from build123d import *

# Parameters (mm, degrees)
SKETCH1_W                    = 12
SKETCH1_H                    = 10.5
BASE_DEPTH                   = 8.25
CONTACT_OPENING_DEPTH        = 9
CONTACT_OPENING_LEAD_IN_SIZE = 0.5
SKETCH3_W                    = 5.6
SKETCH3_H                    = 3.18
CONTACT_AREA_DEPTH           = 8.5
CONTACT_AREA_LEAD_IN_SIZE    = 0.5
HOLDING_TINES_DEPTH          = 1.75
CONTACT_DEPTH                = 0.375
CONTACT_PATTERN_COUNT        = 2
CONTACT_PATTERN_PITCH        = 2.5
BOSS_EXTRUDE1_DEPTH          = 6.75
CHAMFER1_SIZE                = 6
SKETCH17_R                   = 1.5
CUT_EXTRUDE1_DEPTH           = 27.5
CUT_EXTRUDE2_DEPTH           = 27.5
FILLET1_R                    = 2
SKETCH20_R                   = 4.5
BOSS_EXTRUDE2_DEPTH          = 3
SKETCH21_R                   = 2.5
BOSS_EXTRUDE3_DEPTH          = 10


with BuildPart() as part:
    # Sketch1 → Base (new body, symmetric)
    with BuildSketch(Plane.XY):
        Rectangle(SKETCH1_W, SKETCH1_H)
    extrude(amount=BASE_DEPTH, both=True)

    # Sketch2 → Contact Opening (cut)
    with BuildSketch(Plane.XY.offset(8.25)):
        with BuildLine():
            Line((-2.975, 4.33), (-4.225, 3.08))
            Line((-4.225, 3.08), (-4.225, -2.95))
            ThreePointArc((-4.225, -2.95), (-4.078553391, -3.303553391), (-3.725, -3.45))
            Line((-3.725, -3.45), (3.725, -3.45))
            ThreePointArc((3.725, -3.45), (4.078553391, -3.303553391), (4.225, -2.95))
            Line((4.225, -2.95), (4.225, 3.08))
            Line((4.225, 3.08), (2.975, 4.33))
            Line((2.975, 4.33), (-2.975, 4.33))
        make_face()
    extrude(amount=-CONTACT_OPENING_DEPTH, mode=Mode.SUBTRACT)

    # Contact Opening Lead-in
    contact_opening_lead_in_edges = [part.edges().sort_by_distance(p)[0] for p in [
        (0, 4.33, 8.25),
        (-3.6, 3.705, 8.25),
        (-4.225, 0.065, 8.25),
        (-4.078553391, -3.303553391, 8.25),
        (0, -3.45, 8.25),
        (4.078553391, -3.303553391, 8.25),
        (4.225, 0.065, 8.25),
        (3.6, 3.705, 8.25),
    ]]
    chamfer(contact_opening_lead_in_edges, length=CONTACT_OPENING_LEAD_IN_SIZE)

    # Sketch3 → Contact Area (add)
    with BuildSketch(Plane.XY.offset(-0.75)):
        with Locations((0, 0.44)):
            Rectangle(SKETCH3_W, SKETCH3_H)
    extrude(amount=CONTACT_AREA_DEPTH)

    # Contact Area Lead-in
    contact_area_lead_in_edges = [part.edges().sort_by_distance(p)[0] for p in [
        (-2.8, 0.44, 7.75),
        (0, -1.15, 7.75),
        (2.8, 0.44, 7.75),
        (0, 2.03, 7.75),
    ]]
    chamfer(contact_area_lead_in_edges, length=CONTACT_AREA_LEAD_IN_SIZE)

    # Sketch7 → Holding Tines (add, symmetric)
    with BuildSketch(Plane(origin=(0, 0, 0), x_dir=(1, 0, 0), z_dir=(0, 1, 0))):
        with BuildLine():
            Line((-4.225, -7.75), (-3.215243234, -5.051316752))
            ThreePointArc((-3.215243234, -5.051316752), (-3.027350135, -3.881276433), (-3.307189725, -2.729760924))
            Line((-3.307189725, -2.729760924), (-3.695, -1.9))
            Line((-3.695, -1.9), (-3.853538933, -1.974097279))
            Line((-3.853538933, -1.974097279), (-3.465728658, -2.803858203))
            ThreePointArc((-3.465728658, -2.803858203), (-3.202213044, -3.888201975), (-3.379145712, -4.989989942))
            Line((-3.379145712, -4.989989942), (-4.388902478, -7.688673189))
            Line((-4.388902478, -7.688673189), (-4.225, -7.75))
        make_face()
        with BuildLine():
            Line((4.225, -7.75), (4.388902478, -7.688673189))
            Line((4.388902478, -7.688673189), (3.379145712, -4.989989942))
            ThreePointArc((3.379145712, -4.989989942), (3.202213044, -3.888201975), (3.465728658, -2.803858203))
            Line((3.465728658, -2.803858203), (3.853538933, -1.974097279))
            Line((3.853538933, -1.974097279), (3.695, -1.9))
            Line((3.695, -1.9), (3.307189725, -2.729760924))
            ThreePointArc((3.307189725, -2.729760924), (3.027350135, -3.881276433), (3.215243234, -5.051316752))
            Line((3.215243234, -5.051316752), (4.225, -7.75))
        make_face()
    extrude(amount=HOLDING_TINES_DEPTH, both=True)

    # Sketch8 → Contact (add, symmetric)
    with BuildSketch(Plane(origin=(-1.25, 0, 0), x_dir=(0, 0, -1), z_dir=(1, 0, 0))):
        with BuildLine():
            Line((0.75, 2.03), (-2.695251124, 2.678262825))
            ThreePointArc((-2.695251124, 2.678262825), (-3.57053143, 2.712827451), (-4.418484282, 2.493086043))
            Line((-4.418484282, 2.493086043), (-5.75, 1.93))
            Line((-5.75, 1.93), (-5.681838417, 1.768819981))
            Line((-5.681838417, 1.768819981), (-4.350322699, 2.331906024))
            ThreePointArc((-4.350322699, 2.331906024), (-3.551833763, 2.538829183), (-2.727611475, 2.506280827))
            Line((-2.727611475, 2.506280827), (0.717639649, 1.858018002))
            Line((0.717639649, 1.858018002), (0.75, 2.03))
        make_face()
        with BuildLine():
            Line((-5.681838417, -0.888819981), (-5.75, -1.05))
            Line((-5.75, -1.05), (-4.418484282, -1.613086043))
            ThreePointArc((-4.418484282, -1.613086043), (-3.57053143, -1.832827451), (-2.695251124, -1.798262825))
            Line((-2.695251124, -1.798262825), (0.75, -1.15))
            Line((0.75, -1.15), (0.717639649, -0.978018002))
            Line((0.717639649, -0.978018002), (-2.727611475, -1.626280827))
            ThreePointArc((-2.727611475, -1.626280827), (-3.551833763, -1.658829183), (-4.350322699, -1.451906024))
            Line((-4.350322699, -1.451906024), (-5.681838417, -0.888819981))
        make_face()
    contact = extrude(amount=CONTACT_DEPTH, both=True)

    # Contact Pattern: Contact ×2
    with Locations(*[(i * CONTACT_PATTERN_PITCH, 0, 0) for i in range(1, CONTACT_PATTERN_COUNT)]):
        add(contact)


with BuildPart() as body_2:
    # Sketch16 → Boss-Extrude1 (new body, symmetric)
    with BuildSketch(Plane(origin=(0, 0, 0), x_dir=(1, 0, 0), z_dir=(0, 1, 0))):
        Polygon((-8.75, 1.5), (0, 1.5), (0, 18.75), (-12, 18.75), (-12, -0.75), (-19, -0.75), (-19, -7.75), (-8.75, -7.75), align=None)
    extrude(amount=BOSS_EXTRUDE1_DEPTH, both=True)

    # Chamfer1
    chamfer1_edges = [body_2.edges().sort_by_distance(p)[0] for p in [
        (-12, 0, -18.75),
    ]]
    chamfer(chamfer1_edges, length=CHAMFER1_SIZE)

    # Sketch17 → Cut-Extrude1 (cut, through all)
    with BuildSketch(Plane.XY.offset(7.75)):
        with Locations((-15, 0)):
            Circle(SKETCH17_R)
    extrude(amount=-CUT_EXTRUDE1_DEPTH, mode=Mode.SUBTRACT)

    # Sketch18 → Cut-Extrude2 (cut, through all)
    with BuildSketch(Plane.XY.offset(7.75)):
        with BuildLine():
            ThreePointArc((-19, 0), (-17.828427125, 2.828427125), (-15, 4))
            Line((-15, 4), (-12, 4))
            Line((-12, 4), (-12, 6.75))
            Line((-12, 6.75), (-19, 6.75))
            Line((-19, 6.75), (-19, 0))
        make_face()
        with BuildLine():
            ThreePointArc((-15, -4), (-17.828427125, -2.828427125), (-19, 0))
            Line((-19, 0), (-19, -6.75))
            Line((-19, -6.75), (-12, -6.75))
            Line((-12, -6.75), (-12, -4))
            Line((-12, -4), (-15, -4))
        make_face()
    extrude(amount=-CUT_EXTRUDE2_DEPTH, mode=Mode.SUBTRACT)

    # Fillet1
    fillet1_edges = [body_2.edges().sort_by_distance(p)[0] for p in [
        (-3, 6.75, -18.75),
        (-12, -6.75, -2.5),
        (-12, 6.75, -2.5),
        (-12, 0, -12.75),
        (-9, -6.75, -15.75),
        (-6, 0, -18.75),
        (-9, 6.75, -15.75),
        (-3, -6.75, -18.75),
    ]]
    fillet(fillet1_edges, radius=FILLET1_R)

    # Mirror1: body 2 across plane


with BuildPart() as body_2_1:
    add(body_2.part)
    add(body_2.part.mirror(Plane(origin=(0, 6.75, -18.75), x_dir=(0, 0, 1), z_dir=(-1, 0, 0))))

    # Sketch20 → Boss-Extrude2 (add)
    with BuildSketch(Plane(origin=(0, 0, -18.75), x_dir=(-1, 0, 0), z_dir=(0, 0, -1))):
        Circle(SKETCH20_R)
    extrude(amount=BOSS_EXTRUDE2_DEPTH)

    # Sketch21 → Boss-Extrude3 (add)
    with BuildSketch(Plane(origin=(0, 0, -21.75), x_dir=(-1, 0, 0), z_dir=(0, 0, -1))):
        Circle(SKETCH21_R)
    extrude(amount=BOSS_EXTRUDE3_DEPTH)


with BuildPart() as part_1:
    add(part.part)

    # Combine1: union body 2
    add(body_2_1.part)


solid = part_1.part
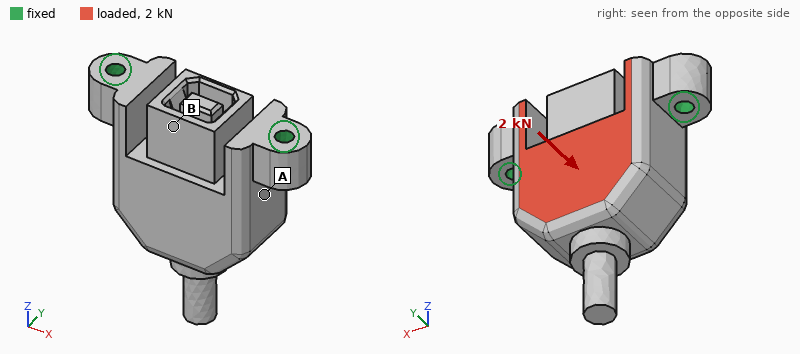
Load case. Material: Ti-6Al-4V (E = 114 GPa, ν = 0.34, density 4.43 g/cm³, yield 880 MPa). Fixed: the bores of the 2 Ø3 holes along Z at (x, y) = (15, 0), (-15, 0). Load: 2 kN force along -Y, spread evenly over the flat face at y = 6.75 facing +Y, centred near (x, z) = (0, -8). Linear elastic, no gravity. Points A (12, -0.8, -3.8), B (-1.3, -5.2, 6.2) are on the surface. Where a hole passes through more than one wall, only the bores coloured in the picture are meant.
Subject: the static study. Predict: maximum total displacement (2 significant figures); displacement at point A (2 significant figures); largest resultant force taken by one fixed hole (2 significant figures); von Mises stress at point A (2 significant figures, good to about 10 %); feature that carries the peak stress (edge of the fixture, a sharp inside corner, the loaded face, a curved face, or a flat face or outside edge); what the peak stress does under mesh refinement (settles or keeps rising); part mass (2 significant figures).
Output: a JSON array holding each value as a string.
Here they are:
["0.12 mm", "0.026 mm", "1.0 kN", "51 MPa", "edge of the fixture", "keeps rising", "34 g"]
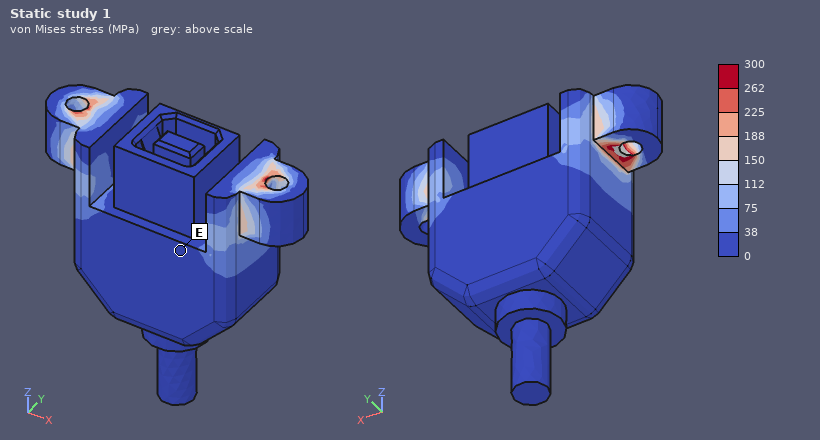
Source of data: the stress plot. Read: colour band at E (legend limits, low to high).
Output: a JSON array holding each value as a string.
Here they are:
["0 to 38 MPa"]
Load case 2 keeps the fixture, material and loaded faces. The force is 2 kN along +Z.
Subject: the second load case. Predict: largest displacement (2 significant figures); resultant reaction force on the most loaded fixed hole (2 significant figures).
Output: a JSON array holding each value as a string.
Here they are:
["74 µm", "1.1 kN"]
